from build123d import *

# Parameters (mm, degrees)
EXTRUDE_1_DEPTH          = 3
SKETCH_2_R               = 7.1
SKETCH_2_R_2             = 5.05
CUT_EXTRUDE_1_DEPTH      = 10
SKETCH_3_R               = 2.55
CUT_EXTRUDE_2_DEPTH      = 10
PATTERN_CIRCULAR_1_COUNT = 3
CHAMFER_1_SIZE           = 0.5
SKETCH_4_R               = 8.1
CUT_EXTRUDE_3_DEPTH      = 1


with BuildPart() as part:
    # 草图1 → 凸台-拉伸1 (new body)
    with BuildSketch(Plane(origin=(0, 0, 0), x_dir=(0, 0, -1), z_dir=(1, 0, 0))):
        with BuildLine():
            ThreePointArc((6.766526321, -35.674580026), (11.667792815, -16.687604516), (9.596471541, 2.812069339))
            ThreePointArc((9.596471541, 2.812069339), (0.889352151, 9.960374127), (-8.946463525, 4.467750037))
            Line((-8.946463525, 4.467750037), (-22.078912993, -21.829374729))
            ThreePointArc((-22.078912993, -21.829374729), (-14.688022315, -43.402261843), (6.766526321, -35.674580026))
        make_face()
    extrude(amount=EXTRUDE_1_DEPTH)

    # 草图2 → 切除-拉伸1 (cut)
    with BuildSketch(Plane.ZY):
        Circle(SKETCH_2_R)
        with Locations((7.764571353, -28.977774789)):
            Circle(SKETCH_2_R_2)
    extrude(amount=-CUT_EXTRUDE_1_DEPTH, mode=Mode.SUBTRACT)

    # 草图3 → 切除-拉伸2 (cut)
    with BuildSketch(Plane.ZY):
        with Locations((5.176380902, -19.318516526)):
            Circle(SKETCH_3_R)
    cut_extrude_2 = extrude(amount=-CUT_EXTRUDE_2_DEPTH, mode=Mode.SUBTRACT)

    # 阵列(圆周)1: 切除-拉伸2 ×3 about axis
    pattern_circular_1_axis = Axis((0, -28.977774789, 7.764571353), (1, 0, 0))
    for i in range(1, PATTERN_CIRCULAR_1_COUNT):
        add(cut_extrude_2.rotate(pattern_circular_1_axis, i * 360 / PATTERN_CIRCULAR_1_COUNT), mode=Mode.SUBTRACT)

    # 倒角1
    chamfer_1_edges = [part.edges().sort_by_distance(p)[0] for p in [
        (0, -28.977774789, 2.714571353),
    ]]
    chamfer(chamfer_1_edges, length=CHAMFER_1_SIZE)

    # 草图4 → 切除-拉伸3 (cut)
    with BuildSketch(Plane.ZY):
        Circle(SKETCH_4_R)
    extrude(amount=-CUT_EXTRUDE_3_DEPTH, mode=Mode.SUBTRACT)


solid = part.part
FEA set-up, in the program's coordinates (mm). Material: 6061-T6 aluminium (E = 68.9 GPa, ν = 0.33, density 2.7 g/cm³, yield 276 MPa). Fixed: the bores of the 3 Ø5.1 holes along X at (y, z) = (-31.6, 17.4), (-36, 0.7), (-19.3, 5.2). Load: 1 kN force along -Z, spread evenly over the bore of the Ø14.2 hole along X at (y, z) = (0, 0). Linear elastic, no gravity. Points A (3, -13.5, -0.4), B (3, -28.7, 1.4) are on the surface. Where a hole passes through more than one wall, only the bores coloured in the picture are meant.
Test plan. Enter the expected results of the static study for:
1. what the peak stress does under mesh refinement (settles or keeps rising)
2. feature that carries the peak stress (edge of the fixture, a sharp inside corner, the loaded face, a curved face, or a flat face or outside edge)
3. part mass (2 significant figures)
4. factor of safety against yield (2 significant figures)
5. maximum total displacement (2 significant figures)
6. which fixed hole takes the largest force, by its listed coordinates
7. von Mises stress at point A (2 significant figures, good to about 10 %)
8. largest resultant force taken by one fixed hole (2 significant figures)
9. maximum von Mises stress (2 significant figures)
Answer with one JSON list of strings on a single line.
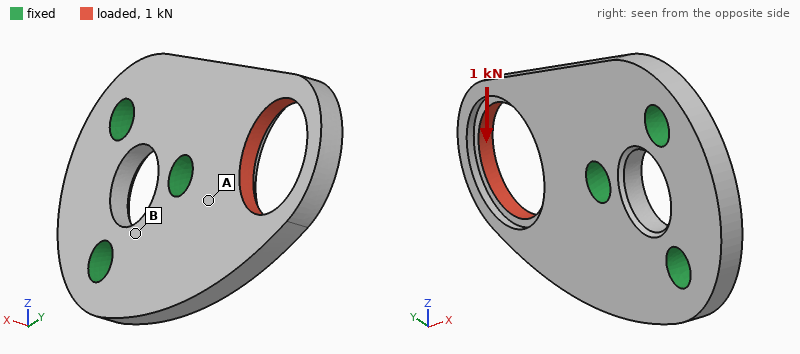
["settles", "the loaded face", "8.9 g", "1.4", "90 µm", "(-19.3, 5.2)", "45 MPa", "1.3 kN", "200 MPa"]
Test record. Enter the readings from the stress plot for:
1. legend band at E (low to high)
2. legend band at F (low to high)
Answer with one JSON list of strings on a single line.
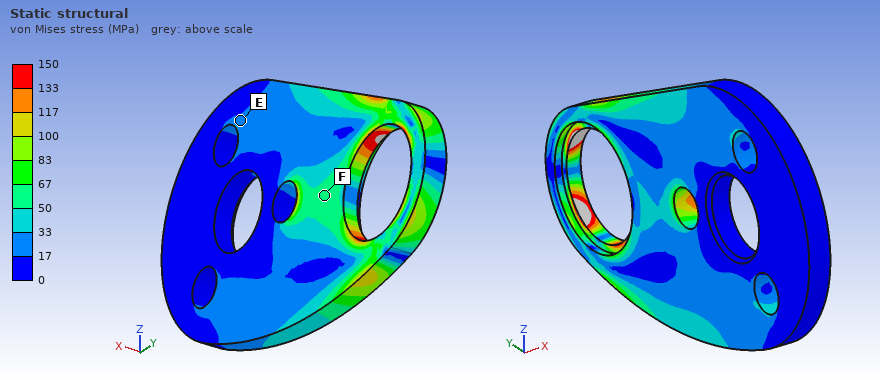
["17 to 33 MPa", "50 to 67 MPa"]
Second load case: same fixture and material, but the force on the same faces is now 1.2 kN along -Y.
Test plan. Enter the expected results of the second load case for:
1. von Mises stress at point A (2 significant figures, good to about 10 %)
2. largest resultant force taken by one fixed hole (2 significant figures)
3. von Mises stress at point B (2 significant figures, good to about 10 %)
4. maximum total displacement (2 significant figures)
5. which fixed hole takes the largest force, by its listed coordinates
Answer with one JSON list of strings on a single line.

["23 MPa", "760 N", "9.1 MPa", "77 µm", "(-19.3, 5.2)"]
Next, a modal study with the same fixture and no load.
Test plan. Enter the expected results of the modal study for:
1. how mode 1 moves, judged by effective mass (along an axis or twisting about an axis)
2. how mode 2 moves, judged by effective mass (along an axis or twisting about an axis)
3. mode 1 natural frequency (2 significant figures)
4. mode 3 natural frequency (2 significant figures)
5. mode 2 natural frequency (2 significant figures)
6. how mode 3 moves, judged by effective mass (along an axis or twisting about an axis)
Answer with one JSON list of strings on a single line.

["along X", "twisting about Y", "4600 Hz", "13 kHz", "7900 Hz", "along X"]
